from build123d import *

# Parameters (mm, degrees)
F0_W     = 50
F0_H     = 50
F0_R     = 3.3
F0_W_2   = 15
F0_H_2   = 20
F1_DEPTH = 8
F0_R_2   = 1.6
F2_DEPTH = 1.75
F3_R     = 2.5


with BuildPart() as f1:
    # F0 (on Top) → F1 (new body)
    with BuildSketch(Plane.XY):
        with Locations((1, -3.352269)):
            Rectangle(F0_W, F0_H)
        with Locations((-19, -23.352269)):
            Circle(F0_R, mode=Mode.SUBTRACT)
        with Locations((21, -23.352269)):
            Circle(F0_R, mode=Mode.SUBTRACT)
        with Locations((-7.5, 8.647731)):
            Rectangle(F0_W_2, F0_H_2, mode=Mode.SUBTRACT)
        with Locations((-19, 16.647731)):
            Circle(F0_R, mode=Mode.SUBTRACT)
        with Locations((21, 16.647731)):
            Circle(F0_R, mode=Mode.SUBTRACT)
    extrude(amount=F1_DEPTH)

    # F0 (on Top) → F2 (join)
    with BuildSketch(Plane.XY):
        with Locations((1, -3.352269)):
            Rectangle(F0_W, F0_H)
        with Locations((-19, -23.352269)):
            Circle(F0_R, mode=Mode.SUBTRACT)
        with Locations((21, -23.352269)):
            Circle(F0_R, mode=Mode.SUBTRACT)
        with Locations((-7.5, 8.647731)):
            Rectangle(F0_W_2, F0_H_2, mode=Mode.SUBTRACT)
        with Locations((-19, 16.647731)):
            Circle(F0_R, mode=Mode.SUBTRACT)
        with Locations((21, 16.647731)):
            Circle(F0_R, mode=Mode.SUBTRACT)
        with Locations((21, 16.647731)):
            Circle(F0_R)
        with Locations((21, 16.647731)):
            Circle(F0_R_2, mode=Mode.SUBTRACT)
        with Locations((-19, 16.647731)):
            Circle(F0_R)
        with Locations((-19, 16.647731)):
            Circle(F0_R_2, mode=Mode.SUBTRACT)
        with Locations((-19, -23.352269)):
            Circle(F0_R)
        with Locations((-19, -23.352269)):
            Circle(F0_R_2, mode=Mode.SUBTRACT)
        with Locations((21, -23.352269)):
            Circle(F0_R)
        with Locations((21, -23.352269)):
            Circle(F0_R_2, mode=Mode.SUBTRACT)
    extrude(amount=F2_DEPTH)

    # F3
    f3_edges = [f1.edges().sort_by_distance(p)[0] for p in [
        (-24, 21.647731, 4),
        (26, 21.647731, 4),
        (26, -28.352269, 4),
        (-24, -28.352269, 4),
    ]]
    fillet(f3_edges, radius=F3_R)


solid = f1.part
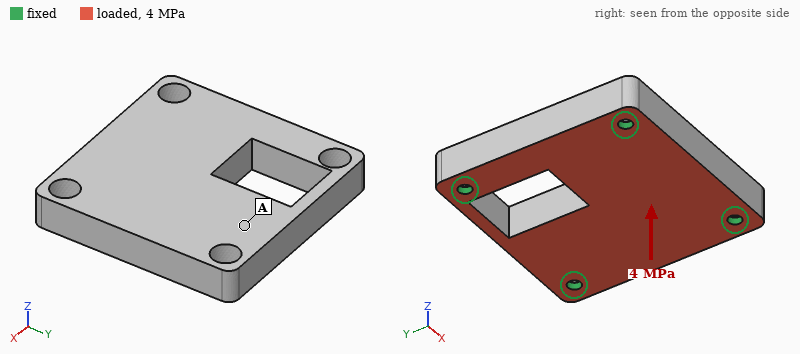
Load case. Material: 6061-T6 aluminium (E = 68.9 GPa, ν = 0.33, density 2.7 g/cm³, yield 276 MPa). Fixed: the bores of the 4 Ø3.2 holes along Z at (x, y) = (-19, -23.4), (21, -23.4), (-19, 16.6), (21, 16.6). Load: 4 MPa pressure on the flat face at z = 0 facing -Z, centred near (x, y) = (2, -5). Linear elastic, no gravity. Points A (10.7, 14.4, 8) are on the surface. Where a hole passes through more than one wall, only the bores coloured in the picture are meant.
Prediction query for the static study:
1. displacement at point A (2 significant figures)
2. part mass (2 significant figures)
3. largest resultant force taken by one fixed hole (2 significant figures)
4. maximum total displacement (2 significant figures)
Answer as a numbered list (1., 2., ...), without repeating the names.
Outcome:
1. 47 µm
2. 45 g
3. 3.1 kN
4. 80 µm
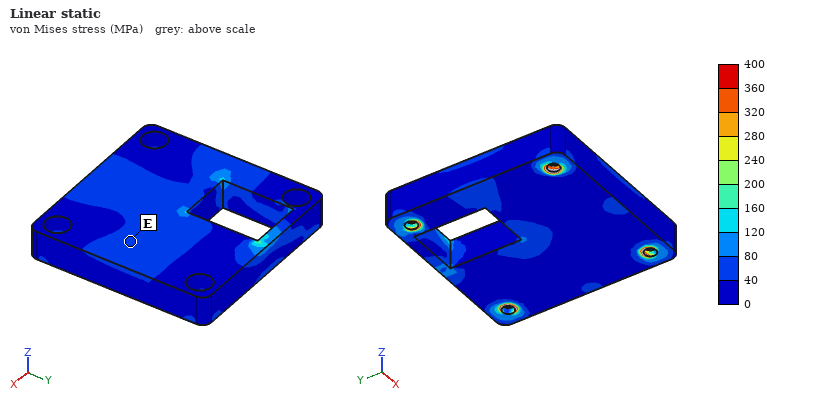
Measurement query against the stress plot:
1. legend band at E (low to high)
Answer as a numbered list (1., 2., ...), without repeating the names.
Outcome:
1. 40 to 80 MPa
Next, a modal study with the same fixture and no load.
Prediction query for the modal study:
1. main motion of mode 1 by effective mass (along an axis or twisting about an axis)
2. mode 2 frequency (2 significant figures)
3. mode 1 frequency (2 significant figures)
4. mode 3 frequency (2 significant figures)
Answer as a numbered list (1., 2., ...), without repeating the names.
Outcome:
1. along Z
2. 15 kHz
3. 9500 Hz
4. 15 kHz
